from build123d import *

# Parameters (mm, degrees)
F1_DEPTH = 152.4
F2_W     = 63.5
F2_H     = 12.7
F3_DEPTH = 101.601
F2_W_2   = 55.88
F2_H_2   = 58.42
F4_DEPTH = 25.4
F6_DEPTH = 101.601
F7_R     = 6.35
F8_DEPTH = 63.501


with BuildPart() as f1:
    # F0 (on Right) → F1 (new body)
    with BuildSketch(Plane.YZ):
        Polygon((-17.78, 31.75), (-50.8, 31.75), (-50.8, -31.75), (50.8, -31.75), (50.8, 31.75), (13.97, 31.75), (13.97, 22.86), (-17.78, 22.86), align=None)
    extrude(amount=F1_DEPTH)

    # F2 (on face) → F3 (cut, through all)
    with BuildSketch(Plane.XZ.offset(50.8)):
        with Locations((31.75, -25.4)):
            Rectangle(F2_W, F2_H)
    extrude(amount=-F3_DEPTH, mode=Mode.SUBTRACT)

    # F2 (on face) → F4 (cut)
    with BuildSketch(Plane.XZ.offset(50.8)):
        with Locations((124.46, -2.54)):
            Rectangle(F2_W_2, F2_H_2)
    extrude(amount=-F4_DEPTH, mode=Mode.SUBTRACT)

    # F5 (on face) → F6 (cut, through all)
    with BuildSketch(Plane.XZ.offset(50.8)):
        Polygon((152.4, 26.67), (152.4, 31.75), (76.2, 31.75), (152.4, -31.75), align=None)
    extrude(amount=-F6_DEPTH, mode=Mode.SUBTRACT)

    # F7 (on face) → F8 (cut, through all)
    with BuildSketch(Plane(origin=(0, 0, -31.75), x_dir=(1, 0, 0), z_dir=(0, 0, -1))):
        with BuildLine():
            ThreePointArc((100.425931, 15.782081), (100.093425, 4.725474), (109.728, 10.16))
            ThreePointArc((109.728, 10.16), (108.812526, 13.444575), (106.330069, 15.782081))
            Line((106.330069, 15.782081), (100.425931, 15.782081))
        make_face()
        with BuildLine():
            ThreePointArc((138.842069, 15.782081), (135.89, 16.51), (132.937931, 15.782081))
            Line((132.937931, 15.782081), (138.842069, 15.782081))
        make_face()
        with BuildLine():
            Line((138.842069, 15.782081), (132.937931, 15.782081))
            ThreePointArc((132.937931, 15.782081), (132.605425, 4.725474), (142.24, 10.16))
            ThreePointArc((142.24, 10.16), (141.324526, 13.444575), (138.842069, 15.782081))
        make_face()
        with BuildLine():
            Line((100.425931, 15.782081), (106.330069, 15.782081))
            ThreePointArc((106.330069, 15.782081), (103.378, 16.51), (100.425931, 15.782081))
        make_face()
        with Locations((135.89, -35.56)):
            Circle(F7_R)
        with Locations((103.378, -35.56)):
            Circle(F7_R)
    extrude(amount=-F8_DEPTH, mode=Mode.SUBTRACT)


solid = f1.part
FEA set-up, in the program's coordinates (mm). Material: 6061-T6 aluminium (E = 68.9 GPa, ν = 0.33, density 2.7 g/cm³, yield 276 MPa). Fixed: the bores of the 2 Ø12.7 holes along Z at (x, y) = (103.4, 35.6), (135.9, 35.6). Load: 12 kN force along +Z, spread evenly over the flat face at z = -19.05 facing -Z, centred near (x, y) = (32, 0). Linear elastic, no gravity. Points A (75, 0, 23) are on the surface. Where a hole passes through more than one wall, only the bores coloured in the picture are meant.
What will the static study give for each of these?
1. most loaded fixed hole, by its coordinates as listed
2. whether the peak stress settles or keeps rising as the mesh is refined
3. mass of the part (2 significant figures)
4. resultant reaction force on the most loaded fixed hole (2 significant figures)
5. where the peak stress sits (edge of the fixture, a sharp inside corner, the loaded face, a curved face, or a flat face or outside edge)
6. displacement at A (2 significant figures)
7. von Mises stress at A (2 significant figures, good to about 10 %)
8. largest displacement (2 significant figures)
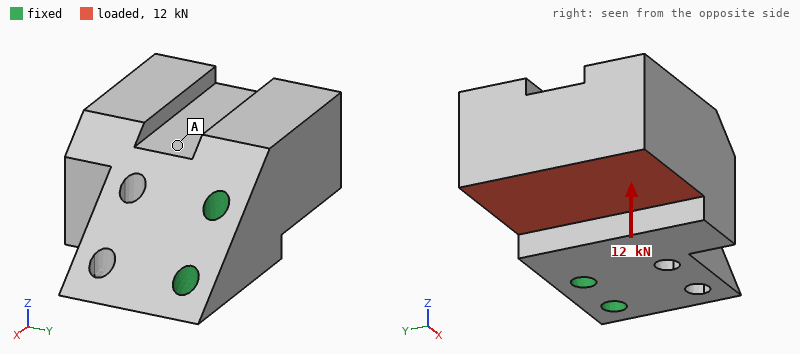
(103.4, 35.6)
keeps rising
1.6 kg
14 kN
edge of the fixture
0.055 mm
11 MPa
0.17 mm
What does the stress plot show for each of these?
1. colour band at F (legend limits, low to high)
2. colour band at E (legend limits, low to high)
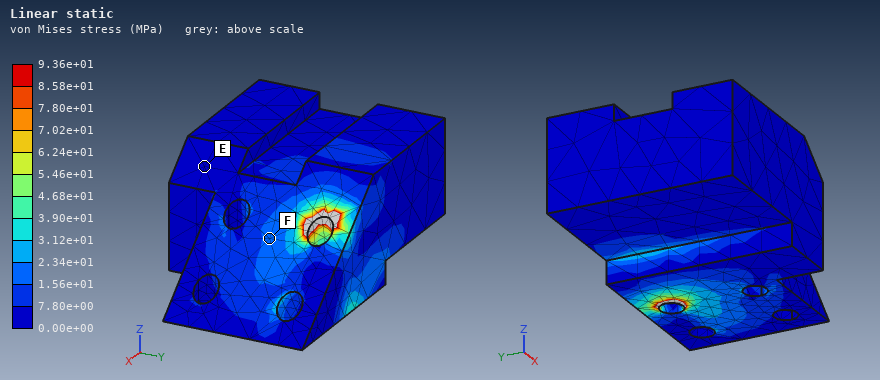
1.56e+01 to 2.34e+01 MPa
0.00e+00 to 7.80e+00 MPa
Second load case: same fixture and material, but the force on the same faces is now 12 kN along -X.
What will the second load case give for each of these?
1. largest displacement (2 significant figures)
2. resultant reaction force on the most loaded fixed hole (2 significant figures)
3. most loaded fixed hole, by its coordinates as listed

72 µm
12 kN
(103.4, 35.6)
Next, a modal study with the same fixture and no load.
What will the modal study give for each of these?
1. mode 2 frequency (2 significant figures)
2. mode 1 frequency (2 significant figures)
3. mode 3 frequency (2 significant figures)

1900 Hz
1500 Hz
3200 Hz
